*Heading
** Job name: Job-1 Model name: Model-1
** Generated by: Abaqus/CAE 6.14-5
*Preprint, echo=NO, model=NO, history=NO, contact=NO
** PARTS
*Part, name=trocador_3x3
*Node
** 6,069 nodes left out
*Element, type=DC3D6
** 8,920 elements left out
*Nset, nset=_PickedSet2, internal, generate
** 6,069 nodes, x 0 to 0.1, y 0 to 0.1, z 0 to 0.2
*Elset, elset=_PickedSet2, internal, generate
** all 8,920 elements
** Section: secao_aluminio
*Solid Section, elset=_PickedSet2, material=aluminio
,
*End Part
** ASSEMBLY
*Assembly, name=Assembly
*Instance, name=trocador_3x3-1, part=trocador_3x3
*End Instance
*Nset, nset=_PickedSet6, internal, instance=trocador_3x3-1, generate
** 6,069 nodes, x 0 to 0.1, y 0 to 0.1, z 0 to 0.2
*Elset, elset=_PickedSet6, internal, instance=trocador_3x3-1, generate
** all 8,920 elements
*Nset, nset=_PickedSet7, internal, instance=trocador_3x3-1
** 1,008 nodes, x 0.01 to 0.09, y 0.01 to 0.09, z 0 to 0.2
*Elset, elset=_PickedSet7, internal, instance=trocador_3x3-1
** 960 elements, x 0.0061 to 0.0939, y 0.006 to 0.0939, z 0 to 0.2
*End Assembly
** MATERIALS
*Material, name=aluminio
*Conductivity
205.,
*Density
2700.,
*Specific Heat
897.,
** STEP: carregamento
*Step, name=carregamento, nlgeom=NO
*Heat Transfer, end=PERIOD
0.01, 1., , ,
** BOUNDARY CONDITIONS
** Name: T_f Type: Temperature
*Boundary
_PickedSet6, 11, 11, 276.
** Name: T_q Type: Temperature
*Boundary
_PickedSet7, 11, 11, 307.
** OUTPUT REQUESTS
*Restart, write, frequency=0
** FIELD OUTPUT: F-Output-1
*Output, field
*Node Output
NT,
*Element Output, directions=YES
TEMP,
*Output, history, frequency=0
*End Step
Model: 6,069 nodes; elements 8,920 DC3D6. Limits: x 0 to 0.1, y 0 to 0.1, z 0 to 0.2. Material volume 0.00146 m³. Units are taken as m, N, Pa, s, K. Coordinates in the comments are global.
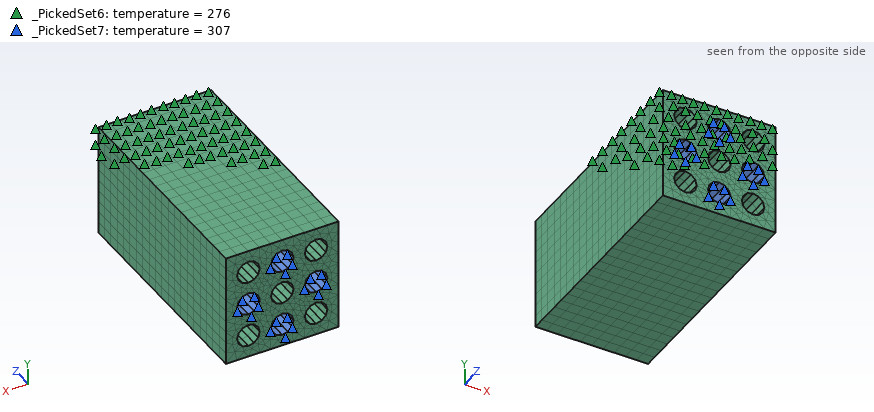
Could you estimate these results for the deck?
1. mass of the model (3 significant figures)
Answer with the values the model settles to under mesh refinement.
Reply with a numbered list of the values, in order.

1. 3.94 kg
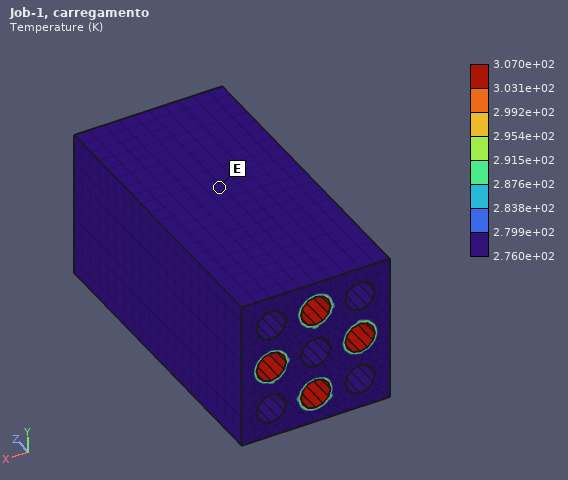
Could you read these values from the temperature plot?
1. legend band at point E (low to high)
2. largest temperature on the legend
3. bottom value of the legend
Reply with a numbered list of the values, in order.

1. 2.760e+02 to 2.799e+02 K
2. 3.070e+02 K
3. 2.760e+02 K
